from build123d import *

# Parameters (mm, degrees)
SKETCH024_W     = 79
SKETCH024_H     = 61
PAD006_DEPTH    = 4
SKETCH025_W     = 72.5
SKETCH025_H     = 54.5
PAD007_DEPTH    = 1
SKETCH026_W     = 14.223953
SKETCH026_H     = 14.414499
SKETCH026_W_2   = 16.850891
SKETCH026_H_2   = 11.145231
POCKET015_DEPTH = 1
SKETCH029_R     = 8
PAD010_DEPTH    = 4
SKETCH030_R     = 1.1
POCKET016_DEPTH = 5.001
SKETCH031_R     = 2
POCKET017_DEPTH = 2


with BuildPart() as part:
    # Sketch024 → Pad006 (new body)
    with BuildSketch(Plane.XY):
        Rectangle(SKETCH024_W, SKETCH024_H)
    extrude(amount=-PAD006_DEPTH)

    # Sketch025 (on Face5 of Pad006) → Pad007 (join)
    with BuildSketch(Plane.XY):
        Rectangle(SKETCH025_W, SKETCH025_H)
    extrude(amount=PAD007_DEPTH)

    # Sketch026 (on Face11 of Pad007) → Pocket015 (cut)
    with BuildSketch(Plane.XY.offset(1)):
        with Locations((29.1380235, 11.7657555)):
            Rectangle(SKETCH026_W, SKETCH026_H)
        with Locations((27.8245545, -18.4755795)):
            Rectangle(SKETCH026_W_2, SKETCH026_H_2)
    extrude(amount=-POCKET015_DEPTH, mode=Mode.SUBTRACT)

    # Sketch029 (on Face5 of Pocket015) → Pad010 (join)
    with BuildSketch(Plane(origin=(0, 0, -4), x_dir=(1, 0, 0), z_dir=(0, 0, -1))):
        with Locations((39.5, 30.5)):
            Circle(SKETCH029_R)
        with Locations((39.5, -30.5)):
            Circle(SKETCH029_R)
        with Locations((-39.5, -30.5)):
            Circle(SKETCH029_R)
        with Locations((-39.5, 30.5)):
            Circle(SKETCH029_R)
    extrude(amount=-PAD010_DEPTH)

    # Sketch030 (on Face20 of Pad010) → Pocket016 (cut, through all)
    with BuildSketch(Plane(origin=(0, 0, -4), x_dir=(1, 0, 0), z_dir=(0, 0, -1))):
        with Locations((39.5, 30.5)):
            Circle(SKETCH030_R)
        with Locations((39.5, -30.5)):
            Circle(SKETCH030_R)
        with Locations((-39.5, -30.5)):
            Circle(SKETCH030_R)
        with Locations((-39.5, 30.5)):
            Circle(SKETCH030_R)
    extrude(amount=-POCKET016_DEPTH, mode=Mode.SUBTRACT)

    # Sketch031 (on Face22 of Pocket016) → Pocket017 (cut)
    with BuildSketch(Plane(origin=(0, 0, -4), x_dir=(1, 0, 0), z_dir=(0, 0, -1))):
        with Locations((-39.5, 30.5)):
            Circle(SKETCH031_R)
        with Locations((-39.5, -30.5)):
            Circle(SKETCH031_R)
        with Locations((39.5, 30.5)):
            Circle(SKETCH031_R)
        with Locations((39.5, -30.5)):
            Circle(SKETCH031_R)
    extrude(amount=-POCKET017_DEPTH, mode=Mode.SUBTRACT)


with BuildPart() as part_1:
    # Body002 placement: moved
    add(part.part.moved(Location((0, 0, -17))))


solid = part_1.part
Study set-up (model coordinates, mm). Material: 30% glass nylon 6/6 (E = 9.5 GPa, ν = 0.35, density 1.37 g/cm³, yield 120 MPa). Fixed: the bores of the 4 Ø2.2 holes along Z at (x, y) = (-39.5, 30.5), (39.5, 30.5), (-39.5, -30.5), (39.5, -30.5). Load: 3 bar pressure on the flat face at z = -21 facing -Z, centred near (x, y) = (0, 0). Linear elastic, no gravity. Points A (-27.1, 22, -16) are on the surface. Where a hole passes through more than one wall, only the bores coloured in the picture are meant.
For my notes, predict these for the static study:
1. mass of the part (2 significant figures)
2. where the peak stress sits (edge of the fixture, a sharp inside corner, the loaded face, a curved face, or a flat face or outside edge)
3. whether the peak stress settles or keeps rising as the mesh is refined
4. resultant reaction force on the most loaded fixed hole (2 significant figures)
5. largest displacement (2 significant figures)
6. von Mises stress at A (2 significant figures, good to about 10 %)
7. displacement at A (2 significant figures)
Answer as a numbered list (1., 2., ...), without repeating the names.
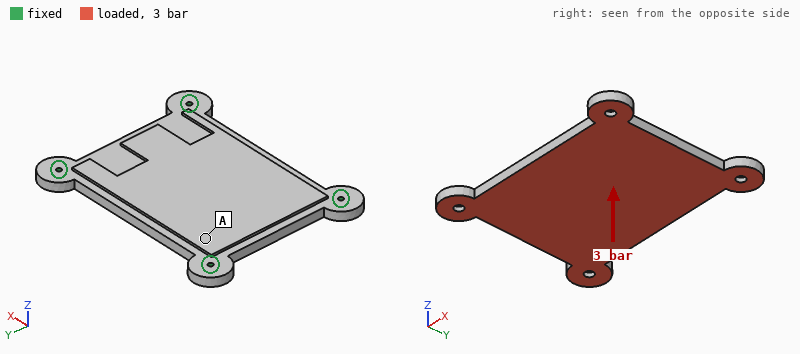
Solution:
1. 34 g
2. edge of the fixture
3. keeps rising
4. 540 N
5. 1.2 mm
6. 24 MPa
7. 0.61 mm
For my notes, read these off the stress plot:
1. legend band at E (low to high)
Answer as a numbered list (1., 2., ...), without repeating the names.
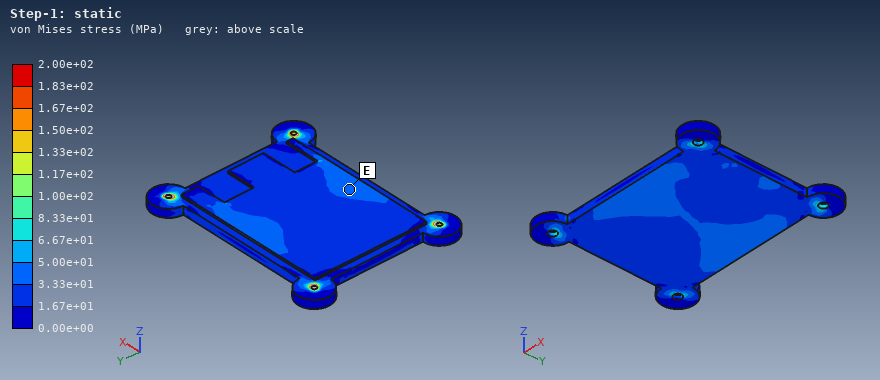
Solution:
1. 3.33e+01 to 5.00e+01 MPa
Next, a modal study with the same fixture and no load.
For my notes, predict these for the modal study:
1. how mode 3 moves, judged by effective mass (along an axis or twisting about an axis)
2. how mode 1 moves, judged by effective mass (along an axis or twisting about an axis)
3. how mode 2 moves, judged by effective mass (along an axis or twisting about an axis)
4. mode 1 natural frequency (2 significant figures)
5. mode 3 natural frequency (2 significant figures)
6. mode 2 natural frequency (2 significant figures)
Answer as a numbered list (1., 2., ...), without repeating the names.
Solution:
1. twisting about Y
2. along Z
3. twisting about X
4. 1100 Hz
5. 2400 Hz
6. 2100 Hz
